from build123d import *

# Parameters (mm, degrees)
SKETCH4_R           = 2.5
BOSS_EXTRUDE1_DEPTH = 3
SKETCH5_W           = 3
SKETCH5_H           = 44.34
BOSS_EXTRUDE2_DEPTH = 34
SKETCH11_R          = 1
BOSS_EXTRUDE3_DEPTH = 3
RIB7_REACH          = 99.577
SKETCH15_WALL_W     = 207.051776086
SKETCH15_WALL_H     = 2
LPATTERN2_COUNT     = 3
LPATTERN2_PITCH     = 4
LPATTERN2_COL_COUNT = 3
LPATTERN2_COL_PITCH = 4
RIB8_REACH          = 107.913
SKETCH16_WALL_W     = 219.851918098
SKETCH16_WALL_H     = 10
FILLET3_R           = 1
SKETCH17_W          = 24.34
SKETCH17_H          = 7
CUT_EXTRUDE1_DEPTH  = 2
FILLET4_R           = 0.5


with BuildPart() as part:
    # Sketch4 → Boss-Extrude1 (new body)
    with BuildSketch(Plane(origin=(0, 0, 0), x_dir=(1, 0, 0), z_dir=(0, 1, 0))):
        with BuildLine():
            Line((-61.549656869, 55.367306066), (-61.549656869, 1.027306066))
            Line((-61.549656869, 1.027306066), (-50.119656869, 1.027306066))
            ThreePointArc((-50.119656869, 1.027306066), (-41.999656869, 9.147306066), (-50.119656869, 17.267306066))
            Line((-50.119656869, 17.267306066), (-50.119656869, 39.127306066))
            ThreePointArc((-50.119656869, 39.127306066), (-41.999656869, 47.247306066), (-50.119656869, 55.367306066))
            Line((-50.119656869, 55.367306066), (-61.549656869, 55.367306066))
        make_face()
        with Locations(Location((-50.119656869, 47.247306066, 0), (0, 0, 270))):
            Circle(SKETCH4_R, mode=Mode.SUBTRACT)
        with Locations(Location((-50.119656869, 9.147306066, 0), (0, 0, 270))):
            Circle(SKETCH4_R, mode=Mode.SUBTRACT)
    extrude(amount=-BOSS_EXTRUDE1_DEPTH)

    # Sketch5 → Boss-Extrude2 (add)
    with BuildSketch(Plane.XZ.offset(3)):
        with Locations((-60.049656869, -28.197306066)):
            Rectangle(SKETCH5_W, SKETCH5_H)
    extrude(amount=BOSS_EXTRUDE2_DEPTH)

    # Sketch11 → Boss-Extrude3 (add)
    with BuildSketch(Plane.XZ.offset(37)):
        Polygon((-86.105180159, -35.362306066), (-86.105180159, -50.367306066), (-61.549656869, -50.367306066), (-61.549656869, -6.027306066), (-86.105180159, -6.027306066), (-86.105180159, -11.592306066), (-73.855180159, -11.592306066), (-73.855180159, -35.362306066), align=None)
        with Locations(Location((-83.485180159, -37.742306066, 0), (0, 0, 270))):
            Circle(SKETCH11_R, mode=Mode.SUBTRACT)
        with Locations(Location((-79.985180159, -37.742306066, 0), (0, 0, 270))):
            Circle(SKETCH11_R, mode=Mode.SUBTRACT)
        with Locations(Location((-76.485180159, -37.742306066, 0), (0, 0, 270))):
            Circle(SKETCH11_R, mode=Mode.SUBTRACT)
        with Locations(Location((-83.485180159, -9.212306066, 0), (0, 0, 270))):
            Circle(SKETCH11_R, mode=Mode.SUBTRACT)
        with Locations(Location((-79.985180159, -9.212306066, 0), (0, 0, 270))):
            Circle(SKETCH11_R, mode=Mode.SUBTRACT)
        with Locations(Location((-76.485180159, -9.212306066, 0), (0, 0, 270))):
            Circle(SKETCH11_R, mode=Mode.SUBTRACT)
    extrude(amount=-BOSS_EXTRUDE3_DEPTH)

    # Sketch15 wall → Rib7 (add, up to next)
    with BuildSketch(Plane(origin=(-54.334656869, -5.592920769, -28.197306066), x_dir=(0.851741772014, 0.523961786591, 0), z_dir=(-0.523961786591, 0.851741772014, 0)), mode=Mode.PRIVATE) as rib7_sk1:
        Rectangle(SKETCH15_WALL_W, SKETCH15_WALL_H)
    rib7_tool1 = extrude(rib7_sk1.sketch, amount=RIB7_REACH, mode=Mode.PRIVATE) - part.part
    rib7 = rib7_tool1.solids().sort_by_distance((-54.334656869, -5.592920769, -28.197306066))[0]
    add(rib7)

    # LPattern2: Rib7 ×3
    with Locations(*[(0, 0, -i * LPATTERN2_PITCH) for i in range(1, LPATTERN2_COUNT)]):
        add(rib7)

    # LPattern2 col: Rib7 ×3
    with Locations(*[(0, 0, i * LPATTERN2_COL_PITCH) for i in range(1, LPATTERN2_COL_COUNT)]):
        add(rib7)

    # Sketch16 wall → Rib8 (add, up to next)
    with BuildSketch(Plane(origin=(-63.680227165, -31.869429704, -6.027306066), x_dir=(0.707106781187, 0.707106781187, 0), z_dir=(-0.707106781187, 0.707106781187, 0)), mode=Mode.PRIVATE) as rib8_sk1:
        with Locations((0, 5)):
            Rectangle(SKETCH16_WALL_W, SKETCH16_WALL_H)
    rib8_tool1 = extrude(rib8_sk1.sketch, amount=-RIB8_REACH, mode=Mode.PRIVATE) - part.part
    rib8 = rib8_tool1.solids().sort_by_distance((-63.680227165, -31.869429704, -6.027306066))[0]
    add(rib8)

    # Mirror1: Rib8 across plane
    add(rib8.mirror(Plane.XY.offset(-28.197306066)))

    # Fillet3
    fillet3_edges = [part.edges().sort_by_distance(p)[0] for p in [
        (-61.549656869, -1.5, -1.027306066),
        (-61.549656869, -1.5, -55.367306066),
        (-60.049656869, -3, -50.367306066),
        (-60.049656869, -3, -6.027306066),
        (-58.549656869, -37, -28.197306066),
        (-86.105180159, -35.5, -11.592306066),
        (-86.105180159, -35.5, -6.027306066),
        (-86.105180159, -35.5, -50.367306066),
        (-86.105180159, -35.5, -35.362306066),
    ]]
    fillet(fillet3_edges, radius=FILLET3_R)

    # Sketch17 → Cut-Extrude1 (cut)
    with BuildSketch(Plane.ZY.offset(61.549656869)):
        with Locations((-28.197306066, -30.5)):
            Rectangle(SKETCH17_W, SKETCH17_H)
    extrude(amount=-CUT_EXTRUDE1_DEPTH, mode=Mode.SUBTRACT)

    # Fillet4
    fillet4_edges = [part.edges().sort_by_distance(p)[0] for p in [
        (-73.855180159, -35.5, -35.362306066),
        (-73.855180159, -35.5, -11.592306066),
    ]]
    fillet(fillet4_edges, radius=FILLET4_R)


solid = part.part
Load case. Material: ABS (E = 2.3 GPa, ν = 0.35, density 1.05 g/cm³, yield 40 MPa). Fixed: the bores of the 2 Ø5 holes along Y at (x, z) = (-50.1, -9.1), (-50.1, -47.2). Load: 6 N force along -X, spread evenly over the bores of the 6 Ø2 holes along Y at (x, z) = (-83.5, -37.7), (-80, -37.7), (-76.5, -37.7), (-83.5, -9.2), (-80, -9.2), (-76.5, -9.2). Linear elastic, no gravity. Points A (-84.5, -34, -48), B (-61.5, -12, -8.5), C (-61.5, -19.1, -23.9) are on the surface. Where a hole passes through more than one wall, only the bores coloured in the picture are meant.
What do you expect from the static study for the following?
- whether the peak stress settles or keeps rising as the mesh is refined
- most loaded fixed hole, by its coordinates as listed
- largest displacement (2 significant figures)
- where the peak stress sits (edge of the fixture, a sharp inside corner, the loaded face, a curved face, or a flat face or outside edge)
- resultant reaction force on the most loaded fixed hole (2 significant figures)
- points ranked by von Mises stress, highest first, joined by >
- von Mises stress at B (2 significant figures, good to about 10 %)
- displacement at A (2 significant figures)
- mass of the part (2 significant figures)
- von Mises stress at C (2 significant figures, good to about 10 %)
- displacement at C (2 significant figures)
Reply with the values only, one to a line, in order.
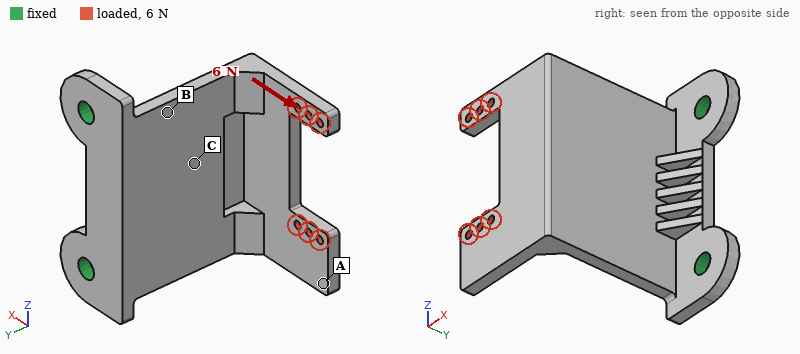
keeps rising
(-50.1, -9.1)
0.80 mm
edge of the fixture
4.4 N
B > C > A
2.2 MPa
0.66 mm
9.7 g
1.2 MPa
0.20 mm
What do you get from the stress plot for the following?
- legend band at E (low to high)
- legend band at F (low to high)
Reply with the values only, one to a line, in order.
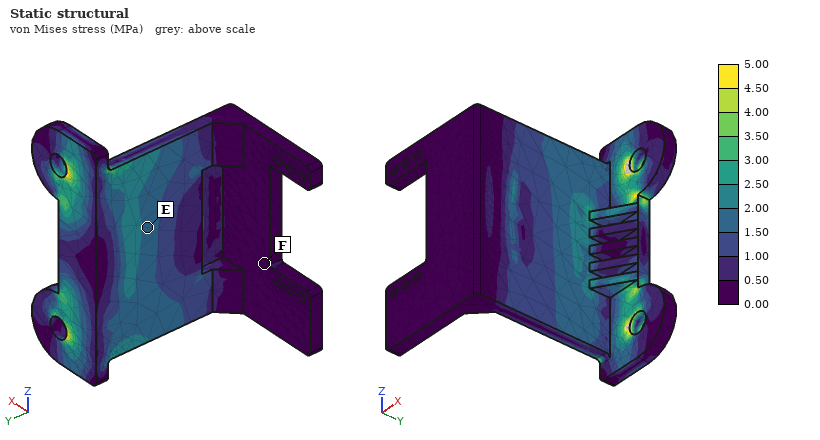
1.50 to 2.00 MPa
0.00 to 0.50 MPa
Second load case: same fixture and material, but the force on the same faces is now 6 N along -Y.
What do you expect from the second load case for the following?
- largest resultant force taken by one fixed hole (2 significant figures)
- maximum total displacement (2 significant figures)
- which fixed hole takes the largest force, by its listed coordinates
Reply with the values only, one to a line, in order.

3.9 N
0.89 mm
(-50.1, -9.1)
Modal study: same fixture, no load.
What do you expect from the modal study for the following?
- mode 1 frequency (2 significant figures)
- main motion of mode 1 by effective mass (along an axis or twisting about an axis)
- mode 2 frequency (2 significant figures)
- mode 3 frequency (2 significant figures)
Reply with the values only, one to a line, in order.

250 Hz
along X
590 Hz
990 Hz
